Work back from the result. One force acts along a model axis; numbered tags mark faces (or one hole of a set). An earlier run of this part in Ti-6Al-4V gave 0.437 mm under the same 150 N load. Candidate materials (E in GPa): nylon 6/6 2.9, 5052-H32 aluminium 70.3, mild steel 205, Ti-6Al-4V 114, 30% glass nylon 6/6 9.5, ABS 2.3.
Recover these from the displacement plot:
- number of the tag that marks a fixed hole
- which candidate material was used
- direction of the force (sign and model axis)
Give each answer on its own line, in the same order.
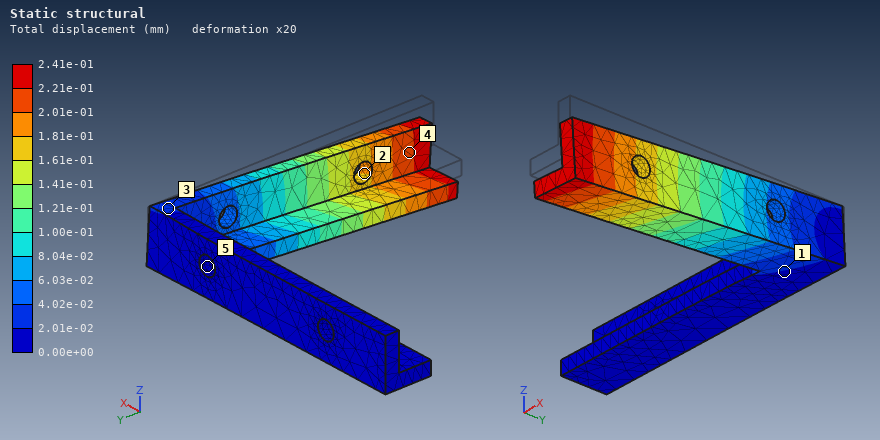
5
mild steel
-Z
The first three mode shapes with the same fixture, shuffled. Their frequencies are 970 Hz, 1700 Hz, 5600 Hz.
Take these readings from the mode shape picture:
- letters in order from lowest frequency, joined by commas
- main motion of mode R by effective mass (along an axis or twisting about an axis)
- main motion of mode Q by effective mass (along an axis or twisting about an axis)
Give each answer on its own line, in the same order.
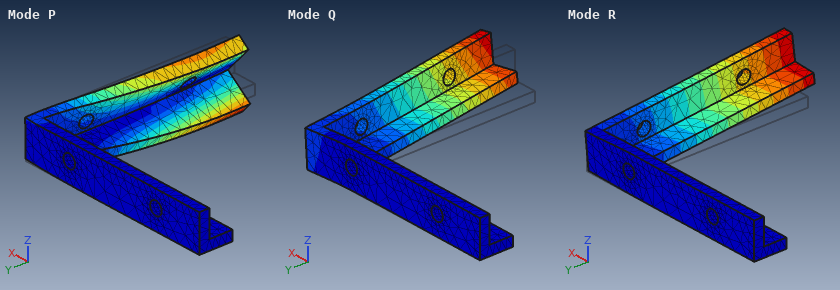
R, Q, P
along Z
along X
